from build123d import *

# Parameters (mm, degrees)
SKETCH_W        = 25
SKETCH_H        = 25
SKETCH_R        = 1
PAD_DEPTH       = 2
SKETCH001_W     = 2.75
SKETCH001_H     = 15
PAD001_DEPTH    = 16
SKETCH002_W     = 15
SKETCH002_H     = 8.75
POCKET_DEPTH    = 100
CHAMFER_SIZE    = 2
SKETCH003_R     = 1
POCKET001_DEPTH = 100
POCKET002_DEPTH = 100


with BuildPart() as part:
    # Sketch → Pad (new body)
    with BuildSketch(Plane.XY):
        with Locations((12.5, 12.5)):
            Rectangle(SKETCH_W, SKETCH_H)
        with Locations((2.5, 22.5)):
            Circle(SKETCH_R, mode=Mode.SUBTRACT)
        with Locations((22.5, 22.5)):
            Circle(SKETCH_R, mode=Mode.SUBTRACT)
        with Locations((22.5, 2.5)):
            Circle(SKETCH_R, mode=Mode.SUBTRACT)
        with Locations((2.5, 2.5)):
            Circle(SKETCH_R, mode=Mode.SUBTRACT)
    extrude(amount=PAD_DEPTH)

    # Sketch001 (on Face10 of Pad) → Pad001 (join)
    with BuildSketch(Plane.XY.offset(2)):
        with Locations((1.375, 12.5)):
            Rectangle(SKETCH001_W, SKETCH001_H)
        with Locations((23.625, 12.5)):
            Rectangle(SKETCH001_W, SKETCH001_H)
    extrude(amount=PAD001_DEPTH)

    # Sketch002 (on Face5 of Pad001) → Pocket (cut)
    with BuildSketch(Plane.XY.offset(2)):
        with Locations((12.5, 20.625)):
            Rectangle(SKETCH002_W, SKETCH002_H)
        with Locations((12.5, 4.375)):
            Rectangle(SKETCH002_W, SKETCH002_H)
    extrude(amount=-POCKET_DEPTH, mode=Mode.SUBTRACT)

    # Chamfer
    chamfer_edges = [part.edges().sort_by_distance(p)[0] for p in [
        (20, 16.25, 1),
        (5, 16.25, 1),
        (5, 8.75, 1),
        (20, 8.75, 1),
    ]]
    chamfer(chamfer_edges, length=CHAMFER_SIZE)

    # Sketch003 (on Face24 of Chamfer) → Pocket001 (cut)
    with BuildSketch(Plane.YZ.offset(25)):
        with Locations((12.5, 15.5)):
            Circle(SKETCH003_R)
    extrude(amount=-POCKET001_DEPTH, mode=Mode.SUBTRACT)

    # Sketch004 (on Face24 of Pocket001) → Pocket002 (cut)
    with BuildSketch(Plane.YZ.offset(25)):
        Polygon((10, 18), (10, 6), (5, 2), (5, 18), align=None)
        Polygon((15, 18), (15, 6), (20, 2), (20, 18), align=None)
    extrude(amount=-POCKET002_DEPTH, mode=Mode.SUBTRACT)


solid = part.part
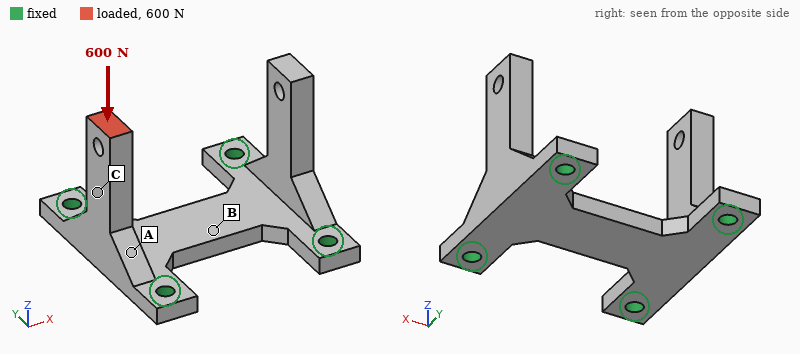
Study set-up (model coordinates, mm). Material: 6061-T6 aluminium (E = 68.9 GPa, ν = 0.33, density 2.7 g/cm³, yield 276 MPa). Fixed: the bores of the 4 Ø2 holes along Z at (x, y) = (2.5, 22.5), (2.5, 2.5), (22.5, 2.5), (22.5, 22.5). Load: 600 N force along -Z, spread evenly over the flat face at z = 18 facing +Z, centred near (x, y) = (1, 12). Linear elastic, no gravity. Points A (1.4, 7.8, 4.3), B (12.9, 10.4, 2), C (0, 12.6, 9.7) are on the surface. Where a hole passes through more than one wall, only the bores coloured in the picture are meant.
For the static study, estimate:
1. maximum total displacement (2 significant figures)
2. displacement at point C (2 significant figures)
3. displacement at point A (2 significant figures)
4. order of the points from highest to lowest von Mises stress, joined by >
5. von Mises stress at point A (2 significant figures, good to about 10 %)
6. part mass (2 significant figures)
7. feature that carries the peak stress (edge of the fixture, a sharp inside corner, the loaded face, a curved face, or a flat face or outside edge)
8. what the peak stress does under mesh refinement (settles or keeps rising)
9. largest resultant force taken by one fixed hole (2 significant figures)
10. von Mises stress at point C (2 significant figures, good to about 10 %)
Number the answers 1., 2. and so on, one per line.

1. 64 µm
2. 41 µm
3. 22 µm
4. A > C > B
5. 100 MPa
6. 3.4 g
7. edge of the fixture
8. keeps rising
9. 380 N
10. 44 MPa
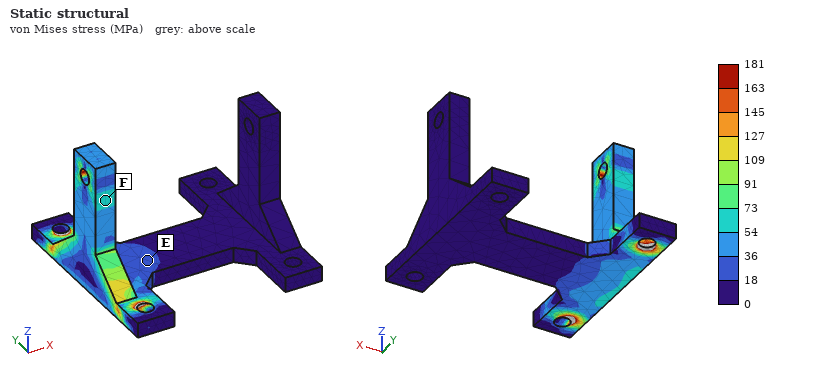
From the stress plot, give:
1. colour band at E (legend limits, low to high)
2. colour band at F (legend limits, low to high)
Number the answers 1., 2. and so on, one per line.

1. 18 to 36 MPa
2. 54 to 73 MPa
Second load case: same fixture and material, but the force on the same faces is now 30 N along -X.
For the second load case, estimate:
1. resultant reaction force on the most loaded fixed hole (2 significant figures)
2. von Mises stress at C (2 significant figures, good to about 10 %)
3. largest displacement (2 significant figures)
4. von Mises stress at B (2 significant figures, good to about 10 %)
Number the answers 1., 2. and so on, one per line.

1. 17 N
2. 40 MPa
3. 0.11 mm
4. 10 MPa
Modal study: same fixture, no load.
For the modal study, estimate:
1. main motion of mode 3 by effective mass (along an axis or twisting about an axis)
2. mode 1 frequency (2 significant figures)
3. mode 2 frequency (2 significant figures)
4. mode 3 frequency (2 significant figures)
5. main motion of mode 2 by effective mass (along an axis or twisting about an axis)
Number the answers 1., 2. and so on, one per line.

1. along Y
2. 6500 Hz
3. 7100 Hz
4. 17 kHz
5. along X
